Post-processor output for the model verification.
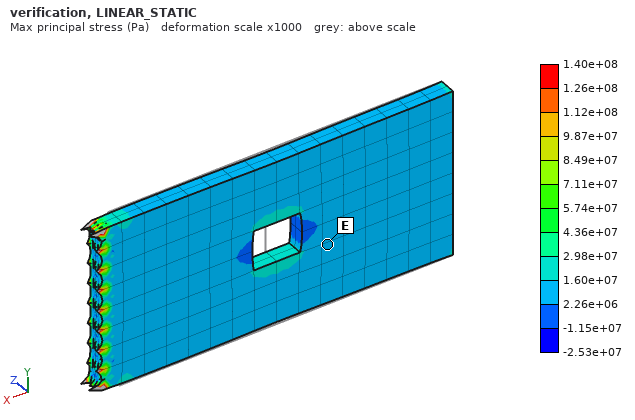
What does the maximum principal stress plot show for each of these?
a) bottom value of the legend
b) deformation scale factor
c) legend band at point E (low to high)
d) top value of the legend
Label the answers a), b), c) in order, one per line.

a) -2.53e+07 Pa
b) 1000
c) 2.26e+06 to 1.60e+07 Pa
d) 1.40e+08 Pa
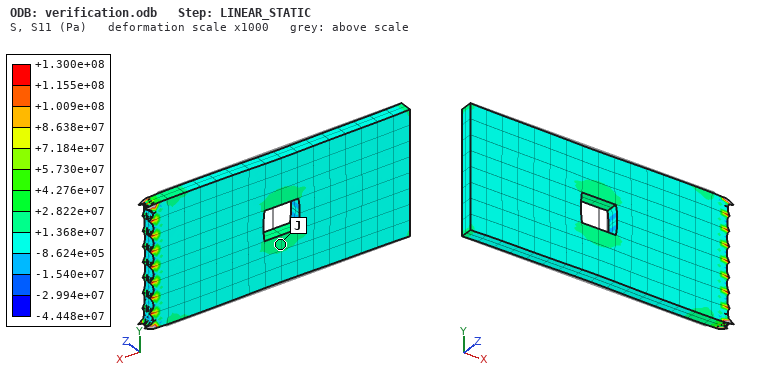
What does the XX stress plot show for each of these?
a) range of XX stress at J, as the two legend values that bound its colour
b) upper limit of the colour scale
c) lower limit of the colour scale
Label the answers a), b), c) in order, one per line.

a) +1.368e+07 to +2.822e+07 Pa
b) +1.300e+08 Pa
c) -4.448e+07 Pa
